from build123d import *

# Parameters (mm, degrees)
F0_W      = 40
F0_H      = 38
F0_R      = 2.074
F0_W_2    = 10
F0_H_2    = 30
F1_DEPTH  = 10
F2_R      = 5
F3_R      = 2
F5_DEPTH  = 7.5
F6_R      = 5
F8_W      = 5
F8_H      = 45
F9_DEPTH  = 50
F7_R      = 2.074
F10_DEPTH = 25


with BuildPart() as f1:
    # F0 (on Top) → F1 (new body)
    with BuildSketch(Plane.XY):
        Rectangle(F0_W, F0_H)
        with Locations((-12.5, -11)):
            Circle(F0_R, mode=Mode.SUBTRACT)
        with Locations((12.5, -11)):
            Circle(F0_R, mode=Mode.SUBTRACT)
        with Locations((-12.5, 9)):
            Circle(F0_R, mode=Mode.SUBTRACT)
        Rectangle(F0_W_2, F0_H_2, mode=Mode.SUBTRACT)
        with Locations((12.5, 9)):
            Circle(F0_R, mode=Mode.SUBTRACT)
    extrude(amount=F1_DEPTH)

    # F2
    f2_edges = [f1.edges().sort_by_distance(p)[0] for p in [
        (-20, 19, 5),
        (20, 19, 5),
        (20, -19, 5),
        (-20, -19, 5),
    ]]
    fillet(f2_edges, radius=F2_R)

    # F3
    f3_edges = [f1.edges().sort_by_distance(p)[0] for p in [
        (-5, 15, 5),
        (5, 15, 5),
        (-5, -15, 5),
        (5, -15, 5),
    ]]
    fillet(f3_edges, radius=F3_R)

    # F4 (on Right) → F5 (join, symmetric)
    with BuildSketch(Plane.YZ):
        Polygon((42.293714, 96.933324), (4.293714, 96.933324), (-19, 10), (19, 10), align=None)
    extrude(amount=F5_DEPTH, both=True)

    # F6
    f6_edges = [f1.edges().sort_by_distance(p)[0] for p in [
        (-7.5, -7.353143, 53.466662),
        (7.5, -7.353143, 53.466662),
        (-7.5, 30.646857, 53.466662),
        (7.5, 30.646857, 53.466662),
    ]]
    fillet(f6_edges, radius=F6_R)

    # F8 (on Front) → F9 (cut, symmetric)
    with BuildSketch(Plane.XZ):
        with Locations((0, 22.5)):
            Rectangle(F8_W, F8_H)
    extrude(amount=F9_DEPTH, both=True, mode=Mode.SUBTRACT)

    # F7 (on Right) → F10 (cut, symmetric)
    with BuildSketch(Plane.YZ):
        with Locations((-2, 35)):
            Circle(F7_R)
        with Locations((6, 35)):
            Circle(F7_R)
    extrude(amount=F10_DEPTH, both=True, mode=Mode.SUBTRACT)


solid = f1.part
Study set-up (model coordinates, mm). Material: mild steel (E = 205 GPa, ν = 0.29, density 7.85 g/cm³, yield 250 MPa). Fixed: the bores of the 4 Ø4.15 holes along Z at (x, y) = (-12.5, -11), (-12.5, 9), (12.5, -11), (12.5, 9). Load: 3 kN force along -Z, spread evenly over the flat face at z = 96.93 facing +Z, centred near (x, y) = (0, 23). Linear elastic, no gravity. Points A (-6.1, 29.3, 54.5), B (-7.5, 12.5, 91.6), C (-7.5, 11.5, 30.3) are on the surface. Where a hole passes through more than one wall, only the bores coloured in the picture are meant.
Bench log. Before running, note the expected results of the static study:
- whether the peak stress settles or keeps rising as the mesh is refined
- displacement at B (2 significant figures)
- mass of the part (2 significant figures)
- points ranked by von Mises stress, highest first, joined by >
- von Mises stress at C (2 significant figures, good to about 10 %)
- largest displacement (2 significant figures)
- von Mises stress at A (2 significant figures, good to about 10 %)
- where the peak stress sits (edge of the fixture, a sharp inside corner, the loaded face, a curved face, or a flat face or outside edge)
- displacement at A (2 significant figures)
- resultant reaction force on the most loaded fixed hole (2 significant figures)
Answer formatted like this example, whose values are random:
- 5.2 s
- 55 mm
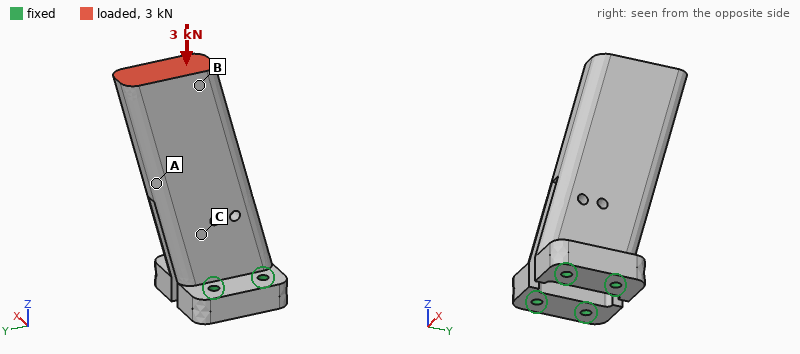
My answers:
- keeps rising
- 39 µm
- 410 g
- C > A > B
- 21 MPa
- 49 µm
- 15 MPa
- edge of the fixture
- 24 µm
- 2.1 kN
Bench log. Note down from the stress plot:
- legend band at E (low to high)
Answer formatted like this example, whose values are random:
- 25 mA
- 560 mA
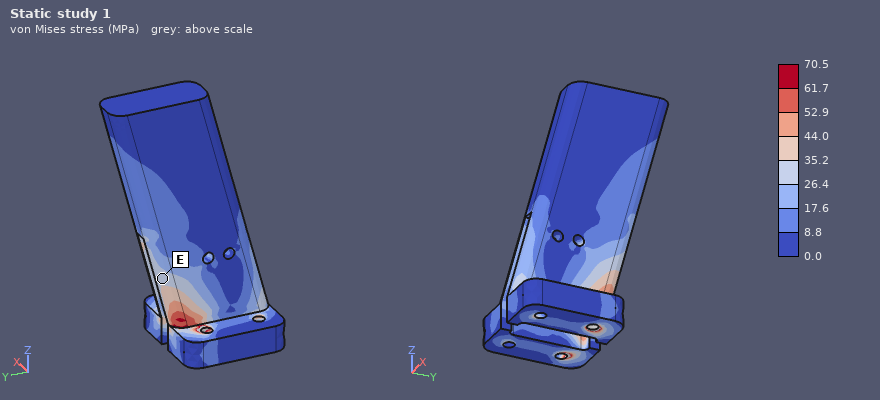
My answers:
- 26.4 to 35.2 MPa
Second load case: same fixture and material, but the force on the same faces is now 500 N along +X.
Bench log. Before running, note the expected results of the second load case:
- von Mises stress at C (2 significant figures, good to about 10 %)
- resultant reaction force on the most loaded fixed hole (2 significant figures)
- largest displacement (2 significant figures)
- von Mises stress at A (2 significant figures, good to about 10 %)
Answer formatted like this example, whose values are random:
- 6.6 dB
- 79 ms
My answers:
- 31 MPa
- 1.7 kN
- 0.11 mm
- 15 MPa
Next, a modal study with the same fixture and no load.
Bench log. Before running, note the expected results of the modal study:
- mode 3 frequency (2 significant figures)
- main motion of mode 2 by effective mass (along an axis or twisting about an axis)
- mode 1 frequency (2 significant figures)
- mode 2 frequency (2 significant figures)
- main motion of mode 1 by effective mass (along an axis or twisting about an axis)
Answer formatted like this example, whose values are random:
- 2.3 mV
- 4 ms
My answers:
- 3200 Hz
- along Y
- 1000 Hz
- 2000 Hz
- along X
